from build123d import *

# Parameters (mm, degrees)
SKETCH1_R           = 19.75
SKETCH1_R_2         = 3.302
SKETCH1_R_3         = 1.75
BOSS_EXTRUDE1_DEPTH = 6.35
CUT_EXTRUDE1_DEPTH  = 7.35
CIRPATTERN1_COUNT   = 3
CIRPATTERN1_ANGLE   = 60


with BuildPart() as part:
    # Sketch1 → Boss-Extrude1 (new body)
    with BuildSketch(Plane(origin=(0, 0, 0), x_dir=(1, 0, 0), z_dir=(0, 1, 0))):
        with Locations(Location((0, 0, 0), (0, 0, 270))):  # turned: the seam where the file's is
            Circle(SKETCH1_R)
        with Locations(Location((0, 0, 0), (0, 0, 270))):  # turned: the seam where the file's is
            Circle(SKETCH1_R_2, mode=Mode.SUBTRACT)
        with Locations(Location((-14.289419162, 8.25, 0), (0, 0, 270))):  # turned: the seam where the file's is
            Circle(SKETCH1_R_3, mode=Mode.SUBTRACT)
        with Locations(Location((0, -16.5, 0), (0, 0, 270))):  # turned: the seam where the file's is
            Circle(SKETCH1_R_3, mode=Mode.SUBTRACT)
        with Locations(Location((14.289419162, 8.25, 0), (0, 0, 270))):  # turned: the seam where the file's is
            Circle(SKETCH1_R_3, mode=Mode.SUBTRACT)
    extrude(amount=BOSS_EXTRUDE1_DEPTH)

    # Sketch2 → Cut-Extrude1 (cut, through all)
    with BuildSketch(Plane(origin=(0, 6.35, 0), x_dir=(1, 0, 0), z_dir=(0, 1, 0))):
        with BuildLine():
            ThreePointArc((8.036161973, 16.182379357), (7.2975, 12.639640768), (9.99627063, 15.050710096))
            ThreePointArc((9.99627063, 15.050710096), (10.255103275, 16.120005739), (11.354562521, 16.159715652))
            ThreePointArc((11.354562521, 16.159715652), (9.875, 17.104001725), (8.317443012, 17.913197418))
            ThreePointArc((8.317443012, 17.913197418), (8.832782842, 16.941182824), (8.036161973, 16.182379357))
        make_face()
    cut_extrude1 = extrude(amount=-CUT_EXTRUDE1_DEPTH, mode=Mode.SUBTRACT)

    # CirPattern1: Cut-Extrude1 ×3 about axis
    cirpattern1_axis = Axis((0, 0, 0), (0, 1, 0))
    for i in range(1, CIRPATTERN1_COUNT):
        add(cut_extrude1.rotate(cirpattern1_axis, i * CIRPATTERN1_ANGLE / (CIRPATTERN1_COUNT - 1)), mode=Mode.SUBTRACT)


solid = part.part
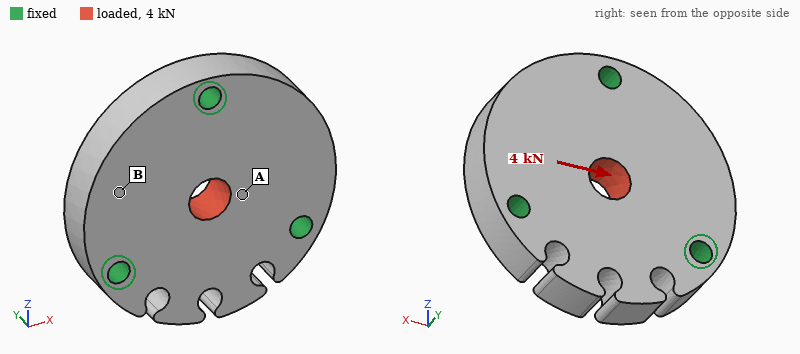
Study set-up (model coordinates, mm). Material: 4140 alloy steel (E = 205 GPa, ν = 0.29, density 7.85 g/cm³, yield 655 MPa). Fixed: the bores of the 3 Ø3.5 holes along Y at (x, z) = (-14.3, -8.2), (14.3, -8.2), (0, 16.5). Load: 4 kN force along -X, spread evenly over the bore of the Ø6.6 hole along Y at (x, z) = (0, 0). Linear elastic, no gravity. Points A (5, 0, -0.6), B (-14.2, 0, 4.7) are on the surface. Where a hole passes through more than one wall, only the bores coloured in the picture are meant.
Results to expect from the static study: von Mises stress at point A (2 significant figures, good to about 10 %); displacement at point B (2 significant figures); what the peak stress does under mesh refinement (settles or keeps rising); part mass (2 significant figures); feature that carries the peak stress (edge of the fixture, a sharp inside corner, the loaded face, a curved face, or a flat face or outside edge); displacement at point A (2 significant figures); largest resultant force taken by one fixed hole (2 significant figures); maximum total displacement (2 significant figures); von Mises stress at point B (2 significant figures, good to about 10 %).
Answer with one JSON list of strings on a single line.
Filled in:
["30 MPa", "1.3 µm", "keeps rising", "56 g", "edge of the fixture", "1.7 µm", "1.4 kN", "2.3 µm", "9.6 MPa"]
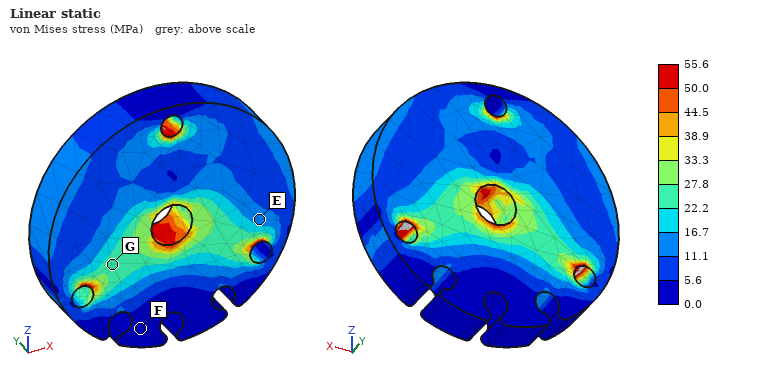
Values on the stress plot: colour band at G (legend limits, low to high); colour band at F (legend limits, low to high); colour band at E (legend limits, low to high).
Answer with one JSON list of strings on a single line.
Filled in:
["22.2 to 27.8 MPa", "0.0 to 5.6 MPa", "11.1 to 16.7 MPa"]
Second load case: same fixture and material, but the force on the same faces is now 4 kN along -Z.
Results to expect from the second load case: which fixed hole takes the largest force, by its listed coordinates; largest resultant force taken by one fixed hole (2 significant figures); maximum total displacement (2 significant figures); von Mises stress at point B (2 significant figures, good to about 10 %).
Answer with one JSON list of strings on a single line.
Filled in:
["(0, 16.5)", "1.6 kN", "2.8 µm", "7.6 MPa"]
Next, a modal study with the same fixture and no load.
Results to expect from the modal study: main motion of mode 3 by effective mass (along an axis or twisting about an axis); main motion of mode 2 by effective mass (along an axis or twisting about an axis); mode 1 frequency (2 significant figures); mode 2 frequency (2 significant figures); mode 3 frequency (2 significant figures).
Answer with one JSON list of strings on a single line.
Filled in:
["along Y", "twisting about Z", "22 kHz", "24 kHz", "26 kHz"]
